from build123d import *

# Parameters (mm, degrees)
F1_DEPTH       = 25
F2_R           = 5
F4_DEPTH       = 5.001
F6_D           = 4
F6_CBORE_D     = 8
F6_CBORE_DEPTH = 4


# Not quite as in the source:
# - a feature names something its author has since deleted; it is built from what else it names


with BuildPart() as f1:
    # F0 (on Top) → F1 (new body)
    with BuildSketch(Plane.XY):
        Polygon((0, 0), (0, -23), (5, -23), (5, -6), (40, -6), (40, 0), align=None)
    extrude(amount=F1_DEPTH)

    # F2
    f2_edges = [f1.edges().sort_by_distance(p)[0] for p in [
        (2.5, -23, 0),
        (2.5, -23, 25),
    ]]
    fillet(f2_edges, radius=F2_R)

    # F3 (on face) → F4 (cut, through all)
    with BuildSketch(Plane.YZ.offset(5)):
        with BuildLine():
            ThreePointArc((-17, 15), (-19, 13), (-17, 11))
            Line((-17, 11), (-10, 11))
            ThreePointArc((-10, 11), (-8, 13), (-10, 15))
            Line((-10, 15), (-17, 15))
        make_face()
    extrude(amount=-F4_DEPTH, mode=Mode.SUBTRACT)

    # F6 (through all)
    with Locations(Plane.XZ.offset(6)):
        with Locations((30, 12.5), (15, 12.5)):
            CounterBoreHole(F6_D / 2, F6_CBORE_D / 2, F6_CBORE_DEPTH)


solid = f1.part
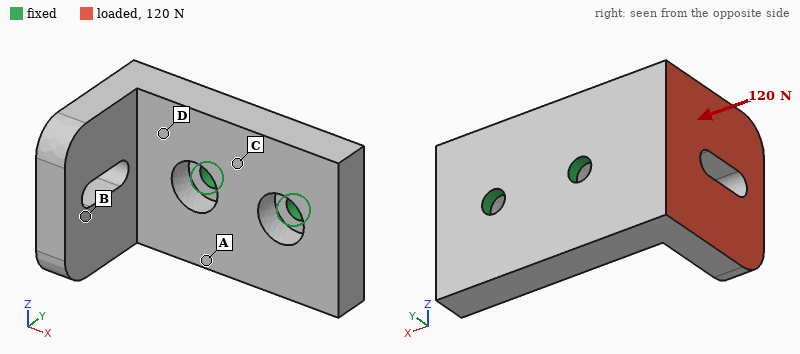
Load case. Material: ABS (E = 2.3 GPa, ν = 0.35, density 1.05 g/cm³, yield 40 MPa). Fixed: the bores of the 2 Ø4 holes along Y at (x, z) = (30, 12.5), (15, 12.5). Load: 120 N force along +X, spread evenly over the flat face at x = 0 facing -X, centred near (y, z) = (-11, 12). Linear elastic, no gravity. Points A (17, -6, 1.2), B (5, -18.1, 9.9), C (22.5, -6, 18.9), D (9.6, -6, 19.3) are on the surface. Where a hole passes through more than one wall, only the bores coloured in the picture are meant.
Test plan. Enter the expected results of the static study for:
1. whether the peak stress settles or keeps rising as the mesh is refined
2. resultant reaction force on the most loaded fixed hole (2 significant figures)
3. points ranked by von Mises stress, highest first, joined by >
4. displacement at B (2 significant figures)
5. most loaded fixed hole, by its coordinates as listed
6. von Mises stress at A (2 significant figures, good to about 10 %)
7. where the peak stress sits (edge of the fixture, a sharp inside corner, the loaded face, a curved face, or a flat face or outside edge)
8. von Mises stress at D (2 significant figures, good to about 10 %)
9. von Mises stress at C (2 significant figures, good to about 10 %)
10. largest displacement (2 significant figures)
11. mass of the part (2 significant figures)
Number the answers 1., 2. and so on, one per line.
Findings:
1. keeps rising
2. 130 N
3. D > A > C > B
4. 0.40 mm
5. (30, 12.5)
6. 6.1 MPa
7. edge of the fixture
8. 8.8 MPa
9. 3.6 MPa
10. 0.58 mm
11. 7.8 g
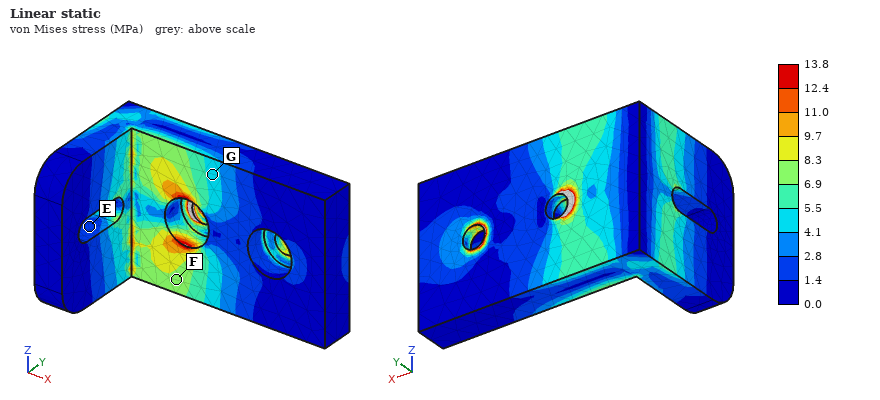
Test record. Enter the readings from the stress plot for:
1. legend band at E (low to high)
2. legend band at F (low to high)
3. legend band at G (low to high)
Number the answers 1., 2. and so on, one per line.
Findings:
1. 1.4 to 2.8 MPa
2. 6.9 to 8.3 MPa
3. 4.1 to 5.5 MPa
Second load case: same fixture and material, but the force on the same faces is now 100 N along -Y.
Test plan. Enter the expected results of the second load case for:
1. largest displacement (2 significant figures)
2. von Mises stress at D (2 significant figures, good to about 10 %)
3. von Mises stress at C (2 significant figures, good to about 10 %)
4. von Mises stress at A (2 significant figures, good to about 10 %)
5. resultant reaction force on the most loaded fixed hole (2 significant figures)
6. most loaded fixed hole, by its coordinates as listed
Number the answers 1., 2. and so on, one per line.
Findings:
1. 0.53 mm
2. 7.8 MPa
3. 4.2 MPa
4. 7.1 MPa
5. 200 N
6. (15, 12.5)
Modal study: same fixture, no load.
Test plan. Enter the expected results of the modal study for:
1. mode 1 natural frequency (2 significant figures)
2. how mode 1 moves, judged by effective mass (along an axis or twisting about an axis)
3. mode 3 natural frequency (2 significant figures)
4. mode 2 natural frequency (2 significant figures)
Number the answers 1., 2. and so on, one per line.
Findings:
1. 1200 Hz
2. along Z
3. 3500 Hz
4. 1400 Hz
